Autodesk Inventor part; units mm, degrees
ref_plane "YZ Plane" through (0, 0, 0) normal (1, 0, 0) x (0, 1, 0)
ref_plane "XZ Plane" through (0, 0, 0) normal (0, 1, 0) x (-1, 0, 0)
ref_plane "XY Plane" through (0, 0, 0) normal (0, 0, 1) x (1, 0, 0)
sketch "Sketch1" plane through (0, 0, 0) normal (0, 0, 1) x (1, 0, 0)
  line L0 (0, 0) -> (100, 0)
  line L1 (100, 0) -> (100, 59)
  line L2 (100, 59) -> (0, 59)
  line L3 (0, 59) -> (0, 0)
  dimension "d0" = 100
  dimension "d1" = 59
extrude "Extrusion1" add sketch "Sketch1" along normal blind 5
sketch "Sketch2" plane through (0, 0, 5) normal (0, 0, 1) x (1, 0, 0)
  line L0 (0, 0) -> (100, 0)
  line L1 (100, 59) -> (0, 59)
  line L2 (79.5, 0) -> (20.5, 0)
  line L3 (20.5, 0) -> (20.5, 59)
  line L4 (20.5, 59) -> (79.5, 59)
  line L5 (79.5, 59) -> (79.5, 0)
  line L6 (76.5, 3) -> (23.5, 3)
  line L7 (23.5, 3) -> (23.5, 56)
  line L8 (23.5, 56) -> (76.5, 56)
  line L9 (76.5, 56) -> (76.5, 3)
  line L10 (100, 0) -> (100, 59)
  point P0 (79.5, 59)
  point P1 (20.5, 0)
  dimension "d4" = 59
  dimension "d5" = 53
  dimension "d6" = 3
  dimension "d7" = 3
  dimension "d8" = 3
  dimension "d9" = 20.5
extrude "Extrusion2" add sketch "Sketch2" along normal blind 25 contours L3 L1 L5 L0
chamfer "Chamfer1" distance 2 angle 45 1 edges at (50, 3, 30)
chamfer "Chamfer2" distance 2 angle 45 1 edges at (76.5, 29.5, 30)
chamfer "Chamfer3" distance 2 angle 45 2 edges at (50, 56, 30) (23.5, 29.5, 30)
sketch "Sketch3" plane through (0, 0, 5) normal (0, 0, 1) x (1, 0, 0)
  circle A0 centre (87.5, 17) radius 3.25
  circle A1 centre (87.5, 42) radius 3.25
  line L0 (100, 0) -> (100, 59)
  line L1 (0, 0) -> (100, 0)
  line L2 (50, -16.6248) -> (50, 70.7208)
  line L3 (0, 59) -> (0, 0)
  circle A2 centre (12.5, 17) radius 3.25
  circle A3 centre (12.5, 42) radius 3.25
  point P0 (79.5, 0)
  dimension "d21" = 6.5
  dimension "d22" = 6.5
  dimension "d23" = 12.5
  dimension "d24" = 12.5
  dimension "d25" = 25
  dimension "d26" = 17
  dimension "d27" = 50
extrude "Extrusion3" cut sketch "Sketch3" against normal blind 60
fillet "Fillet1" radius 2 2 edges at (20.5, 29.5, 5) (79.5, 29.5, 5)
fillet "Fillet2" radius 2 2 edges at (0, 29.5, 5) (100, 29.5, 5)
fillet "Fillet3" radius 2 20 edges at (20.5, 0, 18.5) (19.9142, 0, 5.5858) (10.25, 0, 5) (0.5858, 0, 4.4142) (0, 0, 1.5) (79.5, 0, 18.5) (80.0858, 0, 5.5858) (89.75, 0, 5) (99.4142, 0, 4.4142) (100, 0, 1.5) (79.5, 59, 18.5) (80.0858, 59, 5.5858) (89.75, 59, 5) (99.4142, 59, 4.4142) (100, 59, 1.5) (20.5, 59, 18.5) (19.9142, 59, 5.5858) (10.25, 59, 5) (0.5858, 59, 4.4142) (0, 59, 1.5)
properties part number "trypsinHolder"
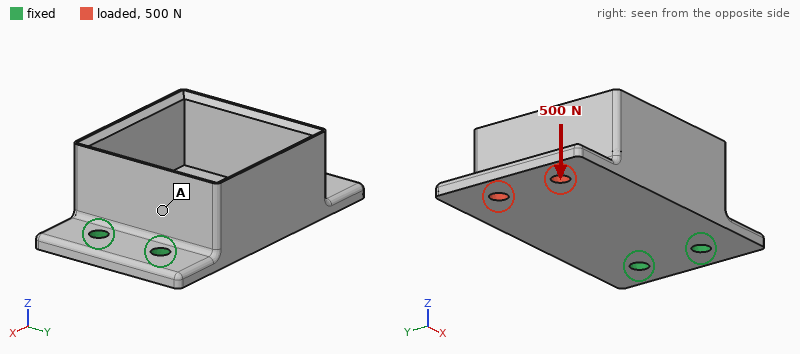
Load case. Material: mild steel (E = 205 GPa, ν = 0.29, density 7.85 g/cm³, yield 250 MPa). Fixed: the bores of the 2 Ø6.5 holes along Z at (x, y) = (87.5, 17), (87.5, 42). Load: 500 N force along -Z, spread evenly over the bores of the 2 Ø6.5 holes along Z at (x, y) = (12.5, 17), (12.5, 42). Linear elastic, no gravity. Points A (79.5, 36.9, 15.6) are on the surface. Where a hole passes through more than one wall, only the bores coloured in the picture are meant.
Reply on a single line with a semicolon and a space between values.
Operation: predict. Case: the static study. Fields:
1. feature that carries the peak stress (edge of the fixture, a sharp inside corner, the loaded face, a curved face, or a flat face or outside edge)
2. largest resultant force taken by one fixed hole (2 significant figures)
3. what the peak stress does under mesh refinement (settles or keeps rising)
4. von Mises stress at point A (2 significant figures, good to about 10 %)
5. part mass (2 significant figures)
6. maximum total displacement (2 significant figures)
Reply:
edge of the fixture; 290 N; keeps rising; 21 MPa; 350 g; 0.30 mm
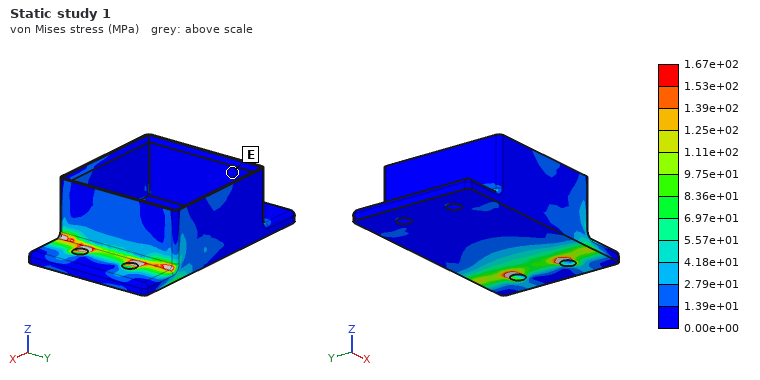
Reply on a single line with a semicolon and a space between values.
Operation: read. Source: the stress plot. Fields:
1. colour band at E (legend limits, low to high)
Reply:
0.00e+00 to 1.39e+01 MPa
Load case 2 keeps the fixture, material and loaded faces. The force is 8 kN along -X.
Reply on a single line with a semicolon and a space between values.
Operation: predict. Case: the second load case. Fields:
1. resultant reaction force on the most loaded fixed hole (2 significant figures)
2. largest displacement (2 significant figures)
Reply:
4.0 kN; 23 µm
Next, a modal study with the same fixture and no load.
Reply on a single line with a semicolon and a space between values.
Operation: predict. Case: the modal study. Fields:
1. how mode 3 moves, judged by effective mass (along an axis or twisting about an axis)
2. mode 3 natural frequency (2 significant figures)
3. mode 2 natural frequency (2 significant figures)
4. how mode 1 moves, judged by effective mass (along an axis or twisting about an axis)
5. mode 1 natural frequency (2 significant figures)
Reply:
along Y; 3300 Hz; 1400 Hz; along Z; 630 Hz
